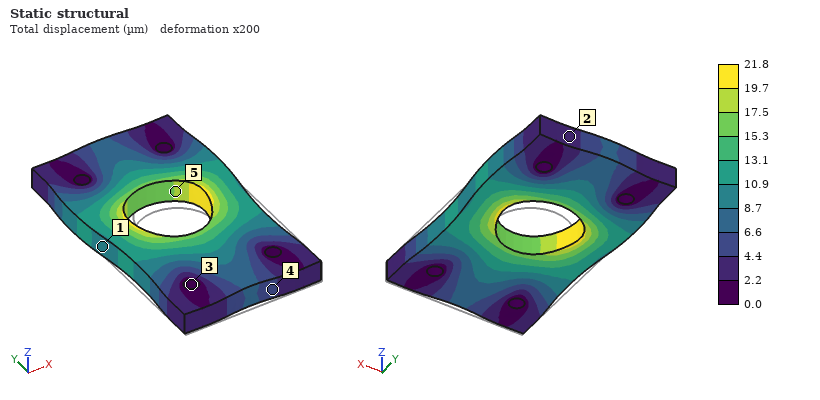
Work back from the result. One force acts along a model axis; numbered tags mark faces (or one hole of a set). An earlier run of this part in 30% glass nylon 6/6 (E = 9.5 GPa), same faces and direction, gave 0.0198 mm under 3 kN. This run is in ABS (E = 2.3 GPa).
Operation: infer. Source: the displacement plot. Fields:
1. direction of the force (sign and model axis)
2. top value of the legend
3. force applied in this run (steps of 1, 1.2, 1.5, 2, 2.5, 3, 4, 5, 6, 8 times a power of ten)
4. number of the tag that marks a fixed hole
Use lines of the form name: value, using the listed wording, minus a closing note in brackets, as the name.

direction of the force: +Y
top value of the legend: 21.8 µm
force applied in this run: 800 N
number of the tag that marks a fixed hole: 3
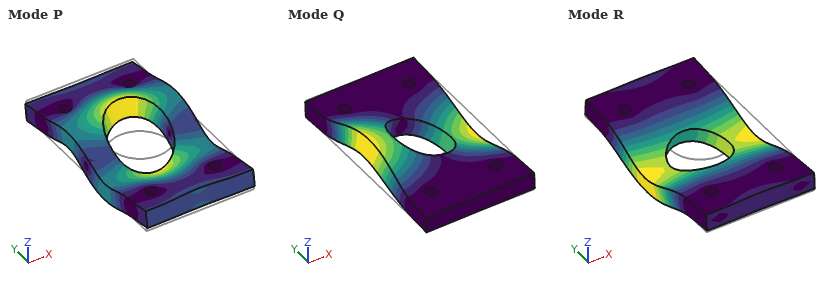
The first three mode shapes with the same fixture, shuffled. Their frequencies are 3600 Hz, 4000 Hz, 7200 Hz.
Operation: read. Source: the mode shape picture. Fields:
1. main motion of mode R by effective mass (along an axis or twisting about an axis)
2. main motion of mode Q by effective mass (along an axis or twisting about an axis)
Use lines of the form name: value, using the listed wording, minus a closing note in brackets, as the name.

main motion of mode R by effective mass: along Z
main motion of mode Q by effective mass: twisting about Y
